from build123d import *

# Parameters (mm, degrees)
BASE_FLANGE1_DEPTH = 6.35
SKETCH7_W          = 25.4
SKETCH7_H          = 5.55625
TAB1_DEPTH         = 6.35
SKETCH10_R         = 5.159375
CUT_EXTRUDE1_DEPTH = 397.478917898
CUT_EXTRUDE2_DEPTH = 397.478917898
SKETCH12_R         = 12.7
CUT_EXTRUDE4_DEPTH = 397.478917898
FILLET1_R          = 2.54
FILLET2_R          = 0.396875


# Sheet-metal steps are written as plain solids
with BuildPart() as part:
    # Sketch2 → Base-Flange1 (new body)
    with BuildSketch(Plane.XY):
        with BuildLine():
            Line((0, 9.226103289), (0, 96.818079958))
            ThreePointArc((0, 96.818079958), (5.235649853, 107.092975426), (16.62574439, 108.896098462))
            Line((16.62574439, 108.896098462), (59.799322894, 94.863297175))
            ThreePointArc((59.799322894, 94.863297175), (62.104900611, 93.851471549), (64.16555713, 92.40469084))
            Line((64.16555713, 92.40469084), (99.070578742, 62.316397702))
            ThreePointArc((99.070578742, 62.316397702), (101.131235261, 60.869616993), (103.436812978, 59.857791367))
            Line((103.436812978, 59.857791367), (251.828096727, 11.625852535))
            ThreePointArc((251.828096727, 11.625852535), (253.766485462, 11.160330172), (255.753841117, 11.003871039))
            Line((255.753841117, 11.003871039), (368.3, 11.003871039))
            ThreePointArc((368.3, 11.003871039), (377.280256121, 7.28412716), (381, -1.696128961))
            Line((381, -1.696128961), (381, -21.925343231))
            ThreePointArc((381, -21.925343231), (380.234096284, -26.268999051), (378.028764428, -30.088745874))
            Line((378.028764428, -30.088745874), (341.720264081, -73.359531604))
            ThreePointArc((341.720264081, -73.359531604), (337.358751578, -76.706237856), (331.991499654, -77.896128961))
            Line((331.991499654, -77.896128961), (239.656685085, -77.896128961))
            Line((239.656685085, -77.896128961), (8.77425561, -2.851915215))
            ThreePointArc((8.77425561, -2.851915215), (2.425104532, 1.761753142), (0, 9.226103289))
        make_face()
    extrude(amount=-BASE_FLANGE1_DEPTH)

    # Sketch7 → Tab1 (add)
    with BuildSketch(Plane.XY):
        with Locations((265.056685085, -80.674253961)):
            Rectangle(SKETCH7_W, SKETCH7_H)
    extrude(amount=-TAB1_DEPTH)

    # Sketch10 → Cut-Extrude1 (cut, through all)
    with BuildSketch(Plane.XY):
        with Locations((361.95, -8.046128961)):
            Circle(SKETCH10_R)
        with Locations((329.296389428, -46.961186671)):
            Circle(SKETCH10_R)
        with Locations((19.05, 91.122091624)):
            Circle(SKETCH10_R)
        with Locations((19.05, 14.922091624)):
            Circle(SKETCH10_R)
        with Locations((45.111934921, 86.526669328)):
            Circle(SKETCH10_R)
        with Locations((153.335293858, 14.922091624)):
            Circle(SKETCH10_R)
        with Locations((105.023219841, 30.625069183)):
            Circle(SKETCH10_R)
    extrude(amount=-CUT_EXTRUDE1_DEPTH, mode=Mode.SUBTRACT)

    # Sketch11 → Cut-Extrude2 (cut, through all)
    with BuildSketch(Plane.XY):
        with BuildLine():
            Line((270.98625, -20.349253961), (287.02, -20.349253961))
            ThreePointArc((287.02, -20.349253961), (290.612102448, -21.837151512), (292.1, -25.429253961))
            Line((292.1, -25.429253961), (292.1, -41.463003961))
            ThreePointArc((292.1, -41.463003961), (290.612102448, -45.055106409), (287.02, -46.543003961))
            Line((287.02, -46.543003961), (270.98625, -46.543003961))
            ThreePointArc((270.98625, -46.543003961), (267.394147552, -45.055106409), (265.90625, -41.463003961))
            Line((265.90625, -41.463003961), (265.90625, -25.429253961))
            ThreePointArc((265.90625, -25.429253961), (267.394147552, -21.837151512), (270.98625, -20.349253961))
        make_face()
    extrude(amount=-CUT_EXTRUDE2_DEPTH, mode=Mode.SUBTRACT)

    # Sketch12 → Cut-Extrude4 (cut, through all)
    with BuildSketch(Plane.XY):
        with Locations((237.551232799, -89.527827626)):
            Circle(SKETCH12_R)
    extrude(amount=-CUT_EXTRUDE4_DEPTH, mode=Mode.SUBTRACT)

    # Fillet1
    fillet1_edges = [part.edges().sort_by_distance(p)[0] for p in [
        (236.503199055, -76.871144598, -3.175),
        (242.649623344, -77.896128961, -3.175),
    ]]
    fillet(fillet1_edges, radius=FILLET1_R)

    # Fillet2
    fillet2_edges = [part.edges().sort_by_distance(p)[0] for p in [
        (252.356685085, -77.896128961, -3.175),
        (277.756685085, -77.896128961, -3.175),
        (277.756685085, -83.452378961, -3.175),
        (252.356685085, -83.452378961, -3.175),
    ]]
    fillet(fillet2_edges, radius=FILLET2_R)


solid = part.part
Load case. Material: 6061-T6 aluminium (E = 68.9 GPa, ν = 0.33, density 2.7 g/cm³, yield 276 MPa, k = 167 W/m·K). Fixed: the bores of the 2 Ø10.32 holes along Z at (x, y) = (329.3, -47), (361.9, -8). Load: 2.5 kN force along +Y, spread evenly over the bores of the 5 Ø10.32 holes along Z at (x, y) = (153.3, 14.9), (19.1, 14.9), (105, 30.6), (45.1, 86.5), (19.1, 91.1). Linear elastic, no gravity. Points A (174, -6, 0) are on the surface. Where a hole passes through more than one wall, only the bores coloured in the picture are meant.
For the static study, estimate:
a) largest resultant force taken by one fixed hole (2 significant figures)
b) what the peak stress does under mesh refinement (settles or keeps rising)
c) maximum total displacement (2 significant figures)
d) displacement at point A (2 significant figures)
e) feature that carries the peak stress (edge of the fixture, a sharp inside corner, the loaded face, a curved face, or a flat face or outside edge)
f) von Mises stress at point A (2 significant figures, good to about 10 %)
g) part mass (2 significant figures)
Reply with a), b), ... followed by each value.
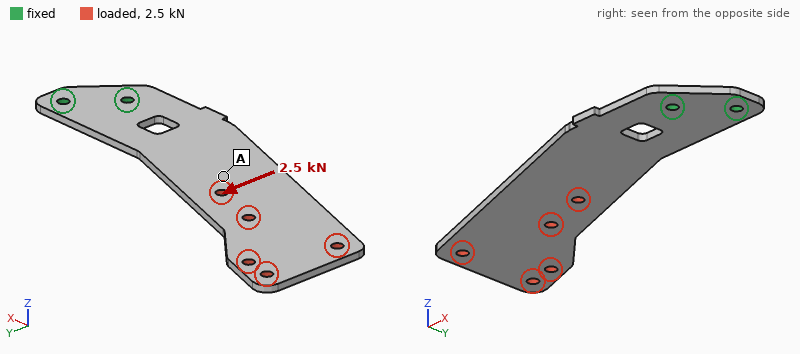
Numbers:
a) 13 kN
b) keeps rising
c) 1.4 mm
d) 0.47 mm
e) edge of the fixture
f) 12 MPa
g) 590 g
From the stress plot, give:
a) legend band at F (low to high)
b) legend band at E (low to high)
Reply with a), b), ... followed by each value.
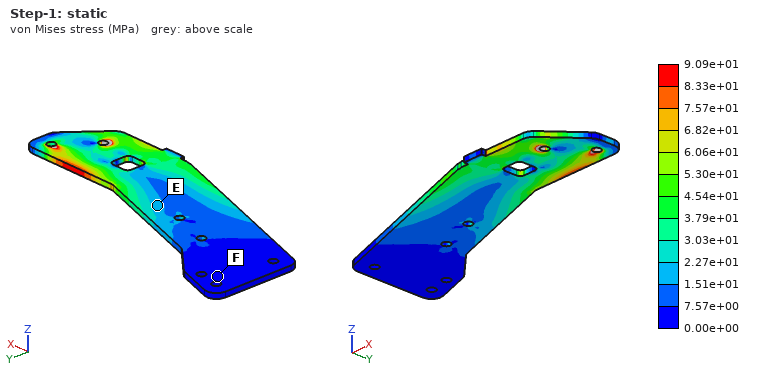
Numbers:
a) 0.00e+00 to 7.57e+00 MPa
b) 1.51e+01 to 2.27e+01 MPa
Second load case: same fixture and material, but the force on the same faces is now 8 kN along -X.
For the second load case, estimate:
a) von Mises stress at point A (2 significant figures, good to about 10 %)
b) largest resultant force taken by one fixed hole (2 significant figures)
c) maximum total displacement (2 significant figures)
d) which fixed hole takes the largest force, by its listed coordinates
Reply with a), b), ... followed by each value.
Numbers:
a) 23 MPa
b) 14 kN
c) 1.7 mm
d) (361.9, -8)
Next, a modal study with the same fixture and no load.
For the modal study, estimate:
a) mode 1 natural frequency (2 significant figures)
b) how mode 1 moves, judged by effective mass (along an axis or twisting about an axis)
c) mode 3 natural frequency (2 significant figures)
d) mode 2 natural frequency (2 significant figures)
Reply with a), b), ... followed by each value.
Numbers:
a) 39 Hz
b) along Z
c) 310 Hz
d) 230 Hz
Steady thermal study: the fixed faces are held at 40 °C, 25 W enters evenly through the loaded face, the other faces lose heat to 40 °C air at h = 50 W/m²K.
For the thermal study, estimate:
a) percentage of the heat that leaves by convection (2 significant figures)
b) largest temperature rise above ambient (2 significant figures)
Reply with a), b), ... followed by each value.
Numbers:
a) 93 %
b) 16 K
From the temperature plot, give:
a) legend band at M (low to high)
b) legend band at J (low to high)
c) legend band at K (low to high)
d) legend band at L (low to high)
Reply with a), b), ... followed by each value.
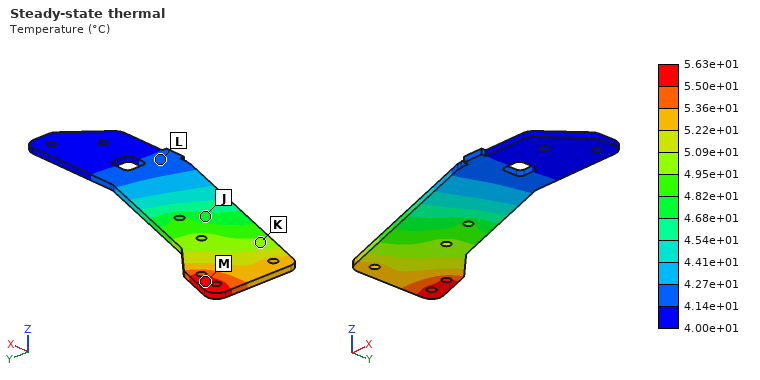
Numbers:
a) 5.50e+01 to 5.63e+01 °C
b) 4.68e+01 to 4.82e+01 °C
c) 4.95e+01 to 5.09e+01 °C
d) 4.14e+01 to 4.27e+01 °C
